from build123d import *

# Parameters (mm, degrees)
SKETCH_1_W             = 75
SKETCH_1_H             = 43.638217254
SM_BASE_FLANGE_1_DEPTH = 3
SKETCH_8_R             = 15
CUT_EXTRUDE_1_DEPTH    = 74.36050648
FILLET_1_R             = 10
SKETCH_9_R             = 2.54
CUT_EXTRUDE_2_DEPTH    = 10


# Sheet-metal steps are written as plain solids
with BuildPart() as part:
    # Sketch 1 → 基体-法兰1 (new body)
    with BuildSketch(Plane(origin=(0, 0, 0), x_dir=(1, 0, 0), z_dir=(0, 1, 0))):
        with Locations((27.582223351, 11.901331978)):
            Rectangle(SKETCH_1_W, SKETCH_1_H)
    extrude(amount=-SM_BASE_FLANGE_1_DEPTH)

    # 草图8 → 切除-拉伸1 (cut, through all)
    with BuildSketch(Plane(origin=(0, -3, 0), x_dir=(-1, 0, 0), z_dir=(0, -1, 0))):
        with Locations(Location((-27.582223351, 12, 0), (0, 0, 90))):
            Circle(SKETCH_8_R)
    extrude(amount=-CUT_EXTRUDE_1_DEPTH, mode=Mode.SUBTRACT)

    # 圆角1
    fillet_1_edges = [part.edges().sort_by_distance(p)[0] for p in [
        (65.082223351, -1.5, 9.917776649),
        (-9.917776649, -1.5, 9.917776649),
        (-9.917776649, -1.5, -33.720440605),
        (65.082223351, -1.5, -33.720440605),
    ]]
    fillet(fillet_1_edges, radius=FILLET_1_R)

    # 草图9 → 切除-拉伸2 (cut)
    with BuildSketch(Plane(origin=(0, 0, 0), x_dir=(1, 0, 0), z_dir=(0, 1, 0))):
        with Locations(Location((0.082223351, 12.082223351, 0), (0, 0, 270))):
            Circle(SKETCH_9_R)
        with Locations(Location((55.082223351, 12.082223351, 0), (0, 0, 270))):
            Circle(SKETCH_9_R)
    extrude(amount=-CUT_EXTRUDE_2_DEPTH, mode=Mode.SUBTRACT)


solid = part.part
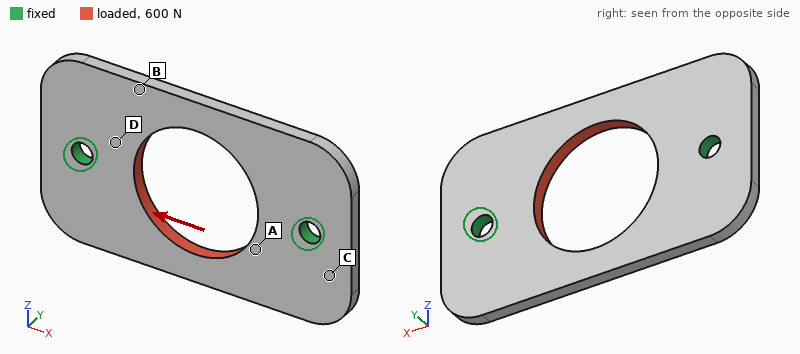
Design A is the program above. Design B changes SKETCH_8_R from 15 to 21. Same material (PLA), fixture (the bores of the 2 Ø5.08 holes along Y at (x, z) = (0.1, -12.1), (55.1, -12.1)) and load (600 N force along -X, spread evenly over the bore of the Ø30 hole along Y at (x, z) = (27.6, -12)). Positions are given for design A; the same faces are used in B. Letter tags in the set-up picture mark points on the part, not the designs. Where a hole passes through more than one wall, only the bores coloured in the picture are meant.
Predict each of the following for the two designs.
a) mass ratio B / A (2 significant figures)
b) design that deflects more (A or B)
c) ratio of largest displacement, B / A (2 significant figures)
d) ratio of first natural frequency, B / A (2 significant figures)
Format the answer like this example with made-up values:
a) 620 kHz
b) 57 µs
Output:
a) 0.72
b) B
c) 3.2
d) 1.1
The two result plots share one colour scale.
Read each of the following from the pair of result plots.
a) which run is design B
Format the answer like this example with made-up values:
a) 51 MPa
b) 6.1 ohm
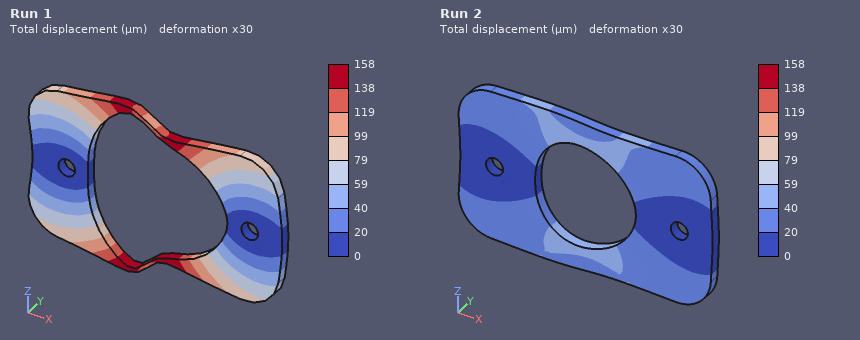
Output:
a) Run 1
